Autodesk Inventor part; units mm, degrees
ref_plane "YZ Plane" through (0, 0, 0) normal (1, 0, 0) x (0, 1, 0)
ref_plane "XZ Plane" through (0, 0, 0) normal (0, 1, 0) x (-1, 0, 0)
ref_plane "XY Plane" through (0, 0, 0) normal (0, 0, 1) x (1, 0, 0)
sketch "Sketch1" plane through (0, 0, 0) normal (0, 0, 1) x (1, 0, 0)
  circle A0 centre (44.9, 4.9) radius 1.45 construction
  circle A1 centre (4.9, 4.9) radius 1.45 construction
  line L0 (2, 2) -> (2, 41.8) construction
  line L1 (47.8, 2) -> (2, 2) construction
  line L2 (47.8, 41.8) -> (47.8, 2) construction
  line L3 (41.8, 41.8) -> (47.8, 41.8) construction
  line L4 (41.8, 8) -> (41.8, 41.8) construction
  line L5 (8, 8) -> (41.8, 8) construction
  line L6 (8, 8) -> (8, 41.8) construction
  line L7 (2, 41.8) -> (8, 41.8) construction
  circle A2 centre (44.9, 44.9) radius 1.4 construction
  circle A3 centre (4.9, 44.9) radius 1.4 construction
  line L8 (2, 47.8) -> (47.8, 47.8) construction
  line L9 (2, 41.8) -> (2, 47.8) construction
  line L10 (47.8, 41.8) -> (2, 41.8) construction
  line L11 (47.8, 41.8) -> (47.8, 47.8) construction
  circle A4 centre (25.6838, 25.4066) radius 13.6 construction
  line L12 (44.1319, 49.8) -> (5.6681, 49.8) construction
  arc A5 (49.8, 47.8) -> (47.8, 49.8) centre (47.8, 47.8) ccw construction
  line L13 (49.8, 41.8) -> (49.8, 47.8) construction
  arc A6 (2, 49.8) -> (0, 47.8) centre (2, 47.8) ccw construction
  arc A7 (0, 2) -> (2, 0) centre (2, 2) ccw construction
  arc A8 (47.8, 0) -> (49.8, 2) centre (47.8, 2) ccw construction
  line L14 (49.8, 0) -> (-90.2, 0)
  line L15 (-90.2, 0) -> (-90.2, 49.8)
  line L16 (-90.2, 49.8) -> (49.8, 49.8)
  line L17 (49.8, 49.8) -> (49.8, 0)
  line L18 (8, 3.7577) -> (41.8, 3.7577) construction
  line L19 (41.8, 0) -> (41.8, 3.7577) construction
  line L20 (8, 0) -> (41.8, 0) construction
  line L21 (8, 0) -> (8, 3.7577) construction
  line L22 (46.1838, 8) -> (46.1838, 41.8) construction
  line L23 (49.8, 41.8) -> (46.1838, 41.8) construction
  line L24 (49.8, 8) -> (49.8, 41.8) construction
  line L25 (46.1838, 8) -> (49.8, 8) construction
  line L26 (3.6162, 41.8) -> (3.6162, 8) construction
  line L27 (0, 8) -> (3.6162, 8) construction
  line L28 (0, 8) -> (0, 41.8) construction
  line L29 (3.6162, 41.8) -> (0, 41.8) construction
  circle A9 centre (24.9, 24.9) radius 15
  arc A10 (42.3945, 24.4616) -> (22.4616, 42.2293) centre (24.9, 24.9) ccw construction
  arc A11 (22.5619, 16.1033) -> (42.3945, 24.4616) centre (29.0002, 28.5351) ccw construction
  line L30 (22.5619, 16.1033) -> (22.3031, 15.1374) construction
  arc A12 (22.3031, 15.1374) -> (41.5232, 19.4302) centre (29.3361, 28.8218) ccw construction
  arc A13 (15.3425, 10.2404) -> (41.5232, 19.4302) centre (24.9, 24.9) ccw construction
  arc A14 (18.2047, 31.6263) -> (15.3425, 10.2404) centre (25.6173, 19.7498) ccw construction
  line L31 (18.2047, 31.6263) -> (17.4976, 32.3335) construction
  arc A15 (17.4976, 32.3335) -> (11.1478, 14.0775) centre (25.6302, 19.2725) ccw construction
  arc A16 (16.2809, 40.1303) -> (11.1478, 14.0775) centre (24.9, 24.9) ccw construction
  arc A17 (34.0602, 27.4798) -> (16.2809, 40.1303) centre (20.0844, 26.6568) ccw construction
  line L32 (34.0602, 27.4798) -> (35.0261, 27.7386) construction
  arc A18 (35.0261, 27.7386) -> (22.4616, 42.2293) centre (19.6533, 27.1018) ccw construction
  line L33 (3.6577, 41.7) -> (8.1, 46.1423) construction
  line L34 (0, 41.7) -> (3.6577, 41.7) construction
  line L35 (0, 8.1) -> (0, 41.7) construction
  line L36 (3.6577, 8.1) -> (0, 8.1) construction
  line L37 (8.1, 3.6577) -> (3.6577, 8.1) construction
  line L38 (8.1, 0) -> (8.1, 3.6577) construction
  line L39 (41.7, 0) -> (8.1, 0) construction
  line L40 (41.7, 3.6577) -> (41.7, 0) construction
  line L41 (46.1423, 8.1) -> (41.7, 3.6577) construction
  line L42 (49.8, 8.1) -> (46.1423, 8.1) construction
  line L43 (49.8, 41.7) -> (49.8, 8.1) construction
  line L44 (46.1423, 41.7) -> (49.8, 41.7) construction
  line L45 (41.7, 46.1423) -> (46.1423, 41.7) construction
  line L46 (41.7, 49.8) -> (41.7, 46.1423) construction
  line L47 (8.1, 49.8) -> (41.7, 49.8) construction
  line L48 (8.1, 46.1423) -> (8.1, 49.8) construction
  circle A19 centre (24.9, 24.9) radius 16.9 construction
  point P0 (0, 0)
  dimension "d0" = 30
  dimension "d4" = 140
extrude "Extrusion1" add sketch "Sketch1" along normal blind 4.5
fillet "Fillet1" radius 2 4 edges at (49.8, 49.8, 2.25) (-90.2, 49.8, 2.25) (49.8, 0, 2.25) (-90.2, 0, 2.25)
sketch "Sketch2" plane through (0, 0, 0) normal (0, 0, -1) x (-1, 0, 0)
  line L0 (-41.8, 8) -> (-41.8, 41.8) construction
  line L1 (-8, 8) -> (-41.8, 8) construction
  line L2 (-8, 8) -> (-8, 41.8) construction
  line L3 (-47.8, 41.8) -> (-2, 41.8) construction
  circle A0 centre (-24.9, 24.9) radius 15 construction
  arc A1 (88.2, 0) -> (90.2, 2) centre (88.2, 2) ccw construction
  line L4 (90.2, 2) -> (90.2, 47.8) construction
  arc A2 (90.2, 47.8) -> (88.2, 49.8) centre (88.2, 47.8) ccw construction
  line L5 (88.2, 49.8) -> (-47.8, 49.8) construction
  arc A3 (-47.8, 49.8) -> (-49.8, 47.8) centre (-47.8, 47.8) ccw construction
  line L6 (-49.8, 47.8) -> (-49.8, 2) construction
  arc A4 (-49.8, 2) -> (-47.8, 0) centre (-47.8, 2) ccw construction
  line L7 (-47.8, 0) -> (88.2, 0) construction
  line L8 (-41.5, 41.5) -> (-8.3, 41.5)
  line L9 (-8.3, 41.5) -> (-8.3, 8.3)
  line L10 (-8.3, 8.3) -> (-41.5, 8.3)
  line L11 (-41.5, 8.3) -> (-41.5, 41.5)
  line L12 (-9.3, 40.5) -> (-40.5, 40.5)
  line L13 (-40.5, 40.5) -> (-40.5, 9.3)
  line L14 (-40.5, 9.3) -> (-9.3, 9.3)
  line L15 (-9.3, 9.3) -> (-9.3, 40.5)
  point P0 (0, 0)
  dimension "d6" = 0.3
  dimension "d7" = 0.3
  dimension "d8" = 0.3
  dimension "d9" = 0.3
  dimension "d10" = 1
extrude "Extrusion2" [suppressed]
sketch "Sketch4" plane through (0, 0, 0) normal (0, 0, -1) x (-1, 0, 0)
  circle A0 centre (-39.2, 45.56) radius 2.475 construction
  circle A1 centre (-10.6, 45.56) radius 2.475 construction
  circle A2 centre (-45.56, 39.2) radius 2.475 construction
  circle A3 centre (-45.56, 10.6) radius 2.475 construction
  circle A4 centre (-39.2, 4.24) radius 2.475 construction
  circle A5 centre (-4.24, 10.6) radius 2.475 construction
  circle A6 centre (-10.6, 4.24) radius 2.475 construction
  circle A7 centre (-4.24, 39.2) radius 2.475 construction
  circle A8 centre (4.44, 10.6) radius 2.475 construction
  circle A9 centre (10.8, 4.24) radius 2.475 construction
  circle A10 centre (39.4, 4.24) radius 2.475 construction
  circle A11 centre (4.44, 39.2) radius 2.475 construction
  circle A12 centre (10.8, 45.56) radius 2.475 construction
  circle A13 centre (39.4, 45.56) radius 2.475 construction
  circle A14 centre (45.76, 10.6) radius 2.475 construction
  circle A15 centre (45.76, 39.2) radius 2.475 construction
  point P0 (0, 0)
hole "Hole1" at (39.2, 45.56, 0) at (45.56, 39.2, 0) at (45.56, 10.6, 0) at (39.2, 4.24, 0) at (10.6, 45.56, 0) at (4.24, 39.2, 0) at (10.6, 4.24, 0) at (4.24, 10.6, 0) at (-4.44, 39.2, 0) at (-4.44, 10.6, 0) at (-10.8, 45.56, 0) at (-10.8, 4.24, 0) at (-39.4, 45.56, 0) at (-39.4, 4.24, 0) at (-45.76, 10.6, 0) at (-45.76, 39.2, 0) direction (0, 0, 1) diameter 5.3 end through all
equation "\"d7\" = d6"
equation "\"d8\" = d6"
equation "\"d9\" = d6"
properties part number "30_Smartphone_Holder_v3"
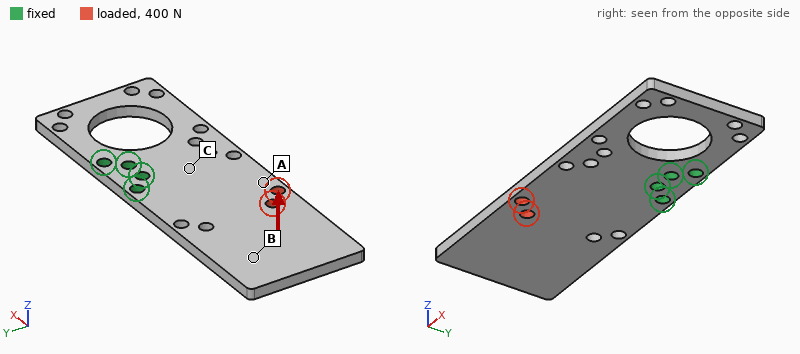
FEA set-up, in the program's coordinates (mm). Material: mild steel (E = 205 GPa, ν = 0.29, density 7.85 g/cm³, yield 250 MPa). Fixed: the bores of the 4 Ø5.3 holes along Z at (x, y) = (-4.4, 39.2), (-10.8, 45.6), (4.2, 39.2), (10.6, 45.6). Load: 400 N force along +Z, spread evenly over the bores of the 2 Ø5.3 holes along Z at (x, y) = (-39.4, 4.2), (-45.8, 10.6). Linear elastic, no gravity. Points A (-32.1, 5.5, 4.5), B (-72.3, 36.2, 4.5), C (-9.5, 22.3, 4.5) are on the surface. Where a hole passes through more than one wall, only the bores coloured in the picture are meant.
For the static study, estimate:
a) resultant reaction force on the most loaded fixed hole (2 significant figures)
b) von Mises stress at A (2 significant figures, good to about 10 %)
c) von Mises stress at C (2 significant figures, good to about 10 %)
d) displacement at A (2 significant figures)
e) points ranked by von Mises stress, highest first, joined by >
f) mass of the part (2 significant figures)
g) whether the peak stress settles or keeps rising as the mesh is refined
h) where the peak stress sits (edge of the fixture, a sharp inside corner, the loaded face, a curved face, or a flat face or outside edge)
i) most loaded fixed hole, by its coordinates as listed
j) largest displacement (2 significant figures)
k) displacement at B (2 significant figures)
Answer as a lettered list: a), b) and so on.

a) 670 N
b) 34 MPa
c) 75 MPa
d) 0.17 mm
e) C > A > B
f) 210 g
g) keeps rising
h) edge of the fixture
i) (-4.4, 39.2)
j) 0.46 mm
k) 0.22 mm
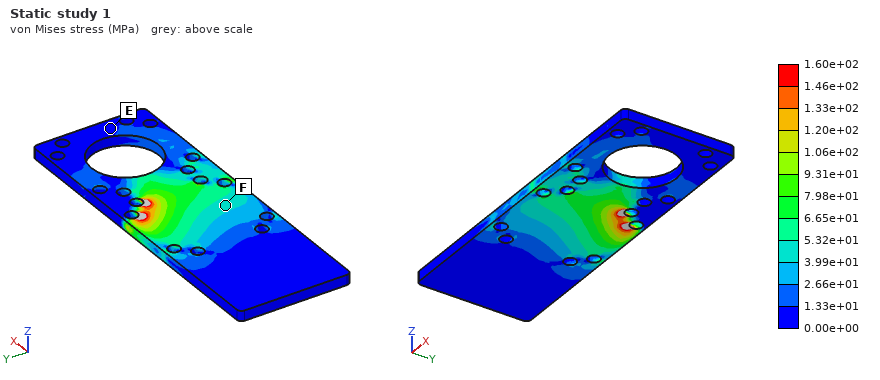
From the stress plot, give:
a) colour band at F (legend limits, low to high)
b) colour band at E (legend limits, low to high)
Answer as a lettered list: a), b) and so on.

a) 3.99e+01 to 5.32e+01 MPa
b) 0.00e+00 to 1.33e+01 MPa
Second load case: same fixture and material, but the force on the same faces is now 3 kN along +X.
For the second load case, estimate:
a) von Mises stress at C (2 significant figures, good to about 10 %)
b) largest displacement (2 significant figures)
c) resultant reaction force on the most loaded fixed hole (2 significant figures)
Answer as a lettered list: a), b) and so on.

a) 43 MPa
b) 69 µm
c) 3.4 kN
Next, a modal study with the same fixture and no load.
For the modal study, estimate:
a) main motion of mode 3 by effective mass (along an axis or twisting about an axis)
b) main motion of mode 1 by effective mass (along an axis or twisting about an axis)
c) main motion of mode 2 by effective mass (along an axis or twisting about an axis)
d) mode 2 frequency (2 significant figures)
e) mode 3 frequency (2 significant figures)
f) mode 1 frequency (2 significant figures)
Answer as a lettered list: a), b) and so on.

a) twisting about X
b) along Z
c) along Z
d) 1300 Hz
e) 1500 Hz
f) 480 Hz
